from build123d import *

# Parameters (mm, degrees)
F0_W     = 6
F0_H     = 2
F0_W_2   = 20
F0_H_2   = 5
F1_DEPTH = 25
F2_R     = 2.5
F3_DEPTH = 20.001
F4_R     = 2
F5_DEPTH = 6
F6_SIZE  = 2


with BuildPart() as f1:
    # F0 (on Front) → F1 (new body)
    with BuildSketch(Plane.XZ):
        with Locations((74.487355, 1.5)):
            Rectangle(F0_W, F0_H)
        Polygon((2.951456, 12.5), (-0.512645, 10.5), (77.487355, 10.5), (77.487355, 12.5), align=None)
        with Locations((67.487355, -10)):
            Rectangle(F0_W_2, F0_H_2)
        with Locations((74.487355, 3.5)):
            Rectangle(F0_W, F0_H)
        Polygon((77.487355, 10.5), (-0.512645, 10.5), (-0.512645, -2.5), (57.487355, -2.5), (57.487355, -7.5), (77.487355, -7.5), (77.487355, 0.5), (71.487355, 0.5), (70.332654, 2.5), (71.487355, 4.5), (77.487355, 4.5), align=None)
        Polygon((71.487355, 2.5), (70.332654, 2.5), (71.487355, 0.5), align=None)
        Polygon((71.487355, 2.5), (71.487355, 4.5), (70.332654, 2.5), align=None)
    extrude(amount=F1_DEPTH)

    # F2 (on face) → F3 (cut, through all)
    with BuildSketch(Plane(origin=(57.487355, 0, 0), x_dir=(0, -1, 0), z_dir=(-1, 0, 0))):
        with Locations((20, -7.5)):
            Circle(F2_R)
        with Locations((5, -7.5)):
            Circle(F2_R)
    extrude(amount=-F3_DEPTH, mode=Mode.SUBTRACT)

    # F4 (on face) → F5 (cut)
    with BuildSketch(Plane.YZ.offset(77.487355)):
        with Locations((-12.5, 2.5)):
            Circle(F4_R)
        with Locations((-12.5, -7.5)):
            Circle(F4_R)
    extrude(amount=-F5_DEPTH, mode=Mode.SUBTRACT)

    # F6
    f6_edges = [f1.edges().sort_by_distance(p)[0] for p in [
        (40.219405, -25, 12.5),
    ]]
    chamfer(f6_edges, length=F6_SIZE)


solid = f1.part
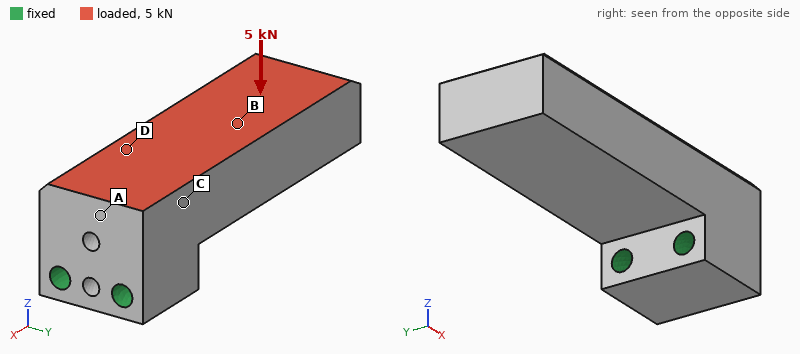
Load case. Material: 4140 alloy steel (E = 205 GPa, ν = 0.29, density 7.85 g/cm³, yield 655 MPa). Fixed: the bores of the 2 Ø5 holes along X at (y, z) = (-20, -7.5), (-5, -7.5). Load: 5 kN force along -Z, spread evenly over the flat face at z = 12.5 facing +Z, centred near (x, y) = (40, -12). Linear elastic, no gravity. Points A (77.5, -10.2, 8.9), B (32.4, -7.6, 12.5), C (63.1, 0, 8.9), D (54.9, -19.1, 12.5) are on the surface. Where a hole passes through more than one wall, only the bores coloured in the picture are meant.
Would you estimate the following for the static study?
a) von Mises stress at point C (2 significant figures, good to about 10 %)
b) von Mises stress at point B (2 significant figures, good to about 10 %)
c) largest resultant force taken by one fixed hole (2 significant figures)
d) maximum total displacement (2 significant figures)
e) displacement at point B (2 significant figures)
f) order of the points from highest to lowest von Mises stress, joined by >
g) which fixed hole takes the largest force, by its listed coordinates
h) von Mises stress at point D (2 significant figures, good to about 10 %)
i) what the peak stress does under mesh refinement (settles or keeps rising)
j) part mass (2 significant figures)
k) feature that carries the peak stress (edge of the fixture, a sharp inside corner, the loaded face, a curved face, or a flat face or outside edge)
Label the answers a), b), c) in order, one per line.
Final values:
a) 57 MPa
b) 33 MPa
c) 2.9 kN
d) 0.12 mm
e) 0.049 mm
f) D > C > B > A
g) (-5, -7.5)
h) 97 MPa
i) keeps rising
j) 260 g
k) a sharp inside corner
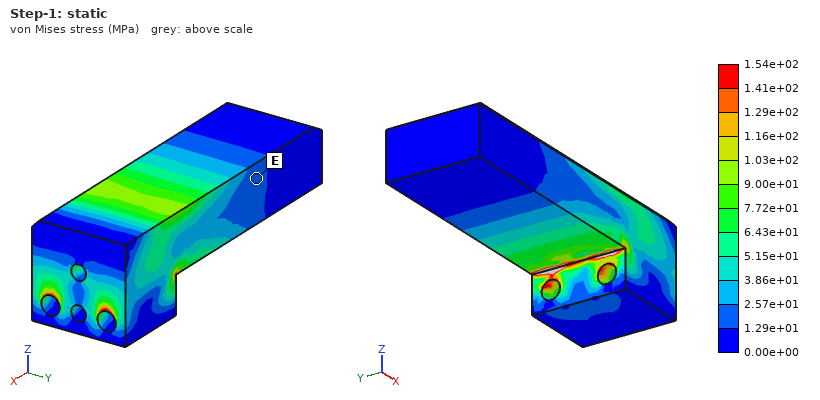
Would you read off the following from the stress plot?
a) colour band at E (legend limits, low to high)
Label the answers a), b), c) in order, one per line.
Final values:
a) 1.29e+01 to 2.57e+01 MPa
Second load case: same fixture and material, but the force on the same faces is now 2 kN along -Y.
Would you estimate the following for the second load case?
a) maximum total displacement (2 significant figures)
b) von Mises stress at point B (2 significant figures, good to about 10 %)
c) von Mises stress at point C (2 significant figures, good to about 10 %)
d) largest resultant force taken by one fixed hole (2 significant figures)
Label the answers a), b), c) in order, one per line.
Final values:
a) 24 µm
b) 13 MPa
c) 15 MPa
d) 3.2 kN
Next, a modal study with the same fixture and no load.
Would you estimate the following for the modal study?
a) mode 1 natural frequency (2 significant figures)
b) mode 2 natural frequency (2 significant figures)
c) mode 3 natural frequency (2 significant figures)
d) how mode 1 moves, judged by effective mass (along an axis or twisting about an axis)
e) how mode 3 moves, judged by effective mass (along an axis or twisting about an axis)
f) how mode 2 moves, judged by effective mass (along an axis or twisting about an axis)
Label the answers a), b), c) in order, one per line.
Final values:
a) 2600 Hz
b) 3600 Hz
c) 10 kHz
d) along Z
e) twisting about X
f) along Y
